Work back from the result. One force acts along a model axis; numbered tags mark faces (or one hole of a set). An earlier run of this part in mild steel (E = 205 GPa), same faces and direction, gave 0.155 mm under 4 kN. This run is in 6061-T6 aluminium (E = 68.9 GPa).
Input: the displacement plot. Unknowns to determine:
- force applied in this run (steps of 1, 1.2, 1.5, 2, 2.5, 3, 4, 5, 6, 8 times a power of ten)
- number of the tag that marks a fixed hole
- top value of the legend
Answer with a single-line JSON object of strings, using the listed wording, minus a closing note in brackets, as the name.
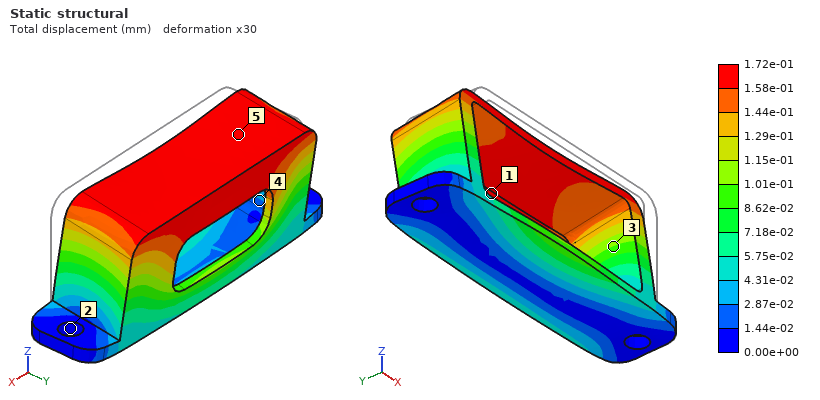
{"force applied in this run": "1.5 kN", "number of the tag that marks a fixed hole": "2", "top value of the legend": "1.72e-01 mm"}
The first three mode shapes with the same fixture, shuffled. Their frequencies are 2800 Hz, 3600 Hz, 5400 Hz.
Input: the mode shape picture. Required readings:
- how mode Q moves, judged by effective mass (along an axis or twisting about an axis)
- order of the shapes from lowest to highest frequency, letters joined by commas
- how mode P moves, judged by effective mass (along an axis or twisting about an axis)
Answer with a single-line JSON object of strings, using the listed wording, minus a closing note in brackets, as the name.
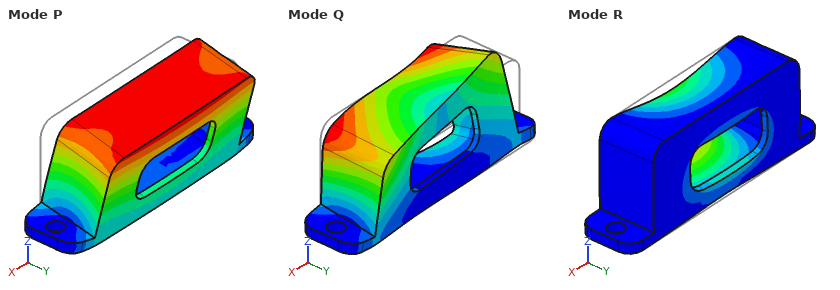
{"how mode Q moves, judged by effective mass": "along X", "order of the shapes from lowest to highest frequency, letters joined by commas": "P, Q, R", "how mode P moves, judged by effective mass": "along Y"}
